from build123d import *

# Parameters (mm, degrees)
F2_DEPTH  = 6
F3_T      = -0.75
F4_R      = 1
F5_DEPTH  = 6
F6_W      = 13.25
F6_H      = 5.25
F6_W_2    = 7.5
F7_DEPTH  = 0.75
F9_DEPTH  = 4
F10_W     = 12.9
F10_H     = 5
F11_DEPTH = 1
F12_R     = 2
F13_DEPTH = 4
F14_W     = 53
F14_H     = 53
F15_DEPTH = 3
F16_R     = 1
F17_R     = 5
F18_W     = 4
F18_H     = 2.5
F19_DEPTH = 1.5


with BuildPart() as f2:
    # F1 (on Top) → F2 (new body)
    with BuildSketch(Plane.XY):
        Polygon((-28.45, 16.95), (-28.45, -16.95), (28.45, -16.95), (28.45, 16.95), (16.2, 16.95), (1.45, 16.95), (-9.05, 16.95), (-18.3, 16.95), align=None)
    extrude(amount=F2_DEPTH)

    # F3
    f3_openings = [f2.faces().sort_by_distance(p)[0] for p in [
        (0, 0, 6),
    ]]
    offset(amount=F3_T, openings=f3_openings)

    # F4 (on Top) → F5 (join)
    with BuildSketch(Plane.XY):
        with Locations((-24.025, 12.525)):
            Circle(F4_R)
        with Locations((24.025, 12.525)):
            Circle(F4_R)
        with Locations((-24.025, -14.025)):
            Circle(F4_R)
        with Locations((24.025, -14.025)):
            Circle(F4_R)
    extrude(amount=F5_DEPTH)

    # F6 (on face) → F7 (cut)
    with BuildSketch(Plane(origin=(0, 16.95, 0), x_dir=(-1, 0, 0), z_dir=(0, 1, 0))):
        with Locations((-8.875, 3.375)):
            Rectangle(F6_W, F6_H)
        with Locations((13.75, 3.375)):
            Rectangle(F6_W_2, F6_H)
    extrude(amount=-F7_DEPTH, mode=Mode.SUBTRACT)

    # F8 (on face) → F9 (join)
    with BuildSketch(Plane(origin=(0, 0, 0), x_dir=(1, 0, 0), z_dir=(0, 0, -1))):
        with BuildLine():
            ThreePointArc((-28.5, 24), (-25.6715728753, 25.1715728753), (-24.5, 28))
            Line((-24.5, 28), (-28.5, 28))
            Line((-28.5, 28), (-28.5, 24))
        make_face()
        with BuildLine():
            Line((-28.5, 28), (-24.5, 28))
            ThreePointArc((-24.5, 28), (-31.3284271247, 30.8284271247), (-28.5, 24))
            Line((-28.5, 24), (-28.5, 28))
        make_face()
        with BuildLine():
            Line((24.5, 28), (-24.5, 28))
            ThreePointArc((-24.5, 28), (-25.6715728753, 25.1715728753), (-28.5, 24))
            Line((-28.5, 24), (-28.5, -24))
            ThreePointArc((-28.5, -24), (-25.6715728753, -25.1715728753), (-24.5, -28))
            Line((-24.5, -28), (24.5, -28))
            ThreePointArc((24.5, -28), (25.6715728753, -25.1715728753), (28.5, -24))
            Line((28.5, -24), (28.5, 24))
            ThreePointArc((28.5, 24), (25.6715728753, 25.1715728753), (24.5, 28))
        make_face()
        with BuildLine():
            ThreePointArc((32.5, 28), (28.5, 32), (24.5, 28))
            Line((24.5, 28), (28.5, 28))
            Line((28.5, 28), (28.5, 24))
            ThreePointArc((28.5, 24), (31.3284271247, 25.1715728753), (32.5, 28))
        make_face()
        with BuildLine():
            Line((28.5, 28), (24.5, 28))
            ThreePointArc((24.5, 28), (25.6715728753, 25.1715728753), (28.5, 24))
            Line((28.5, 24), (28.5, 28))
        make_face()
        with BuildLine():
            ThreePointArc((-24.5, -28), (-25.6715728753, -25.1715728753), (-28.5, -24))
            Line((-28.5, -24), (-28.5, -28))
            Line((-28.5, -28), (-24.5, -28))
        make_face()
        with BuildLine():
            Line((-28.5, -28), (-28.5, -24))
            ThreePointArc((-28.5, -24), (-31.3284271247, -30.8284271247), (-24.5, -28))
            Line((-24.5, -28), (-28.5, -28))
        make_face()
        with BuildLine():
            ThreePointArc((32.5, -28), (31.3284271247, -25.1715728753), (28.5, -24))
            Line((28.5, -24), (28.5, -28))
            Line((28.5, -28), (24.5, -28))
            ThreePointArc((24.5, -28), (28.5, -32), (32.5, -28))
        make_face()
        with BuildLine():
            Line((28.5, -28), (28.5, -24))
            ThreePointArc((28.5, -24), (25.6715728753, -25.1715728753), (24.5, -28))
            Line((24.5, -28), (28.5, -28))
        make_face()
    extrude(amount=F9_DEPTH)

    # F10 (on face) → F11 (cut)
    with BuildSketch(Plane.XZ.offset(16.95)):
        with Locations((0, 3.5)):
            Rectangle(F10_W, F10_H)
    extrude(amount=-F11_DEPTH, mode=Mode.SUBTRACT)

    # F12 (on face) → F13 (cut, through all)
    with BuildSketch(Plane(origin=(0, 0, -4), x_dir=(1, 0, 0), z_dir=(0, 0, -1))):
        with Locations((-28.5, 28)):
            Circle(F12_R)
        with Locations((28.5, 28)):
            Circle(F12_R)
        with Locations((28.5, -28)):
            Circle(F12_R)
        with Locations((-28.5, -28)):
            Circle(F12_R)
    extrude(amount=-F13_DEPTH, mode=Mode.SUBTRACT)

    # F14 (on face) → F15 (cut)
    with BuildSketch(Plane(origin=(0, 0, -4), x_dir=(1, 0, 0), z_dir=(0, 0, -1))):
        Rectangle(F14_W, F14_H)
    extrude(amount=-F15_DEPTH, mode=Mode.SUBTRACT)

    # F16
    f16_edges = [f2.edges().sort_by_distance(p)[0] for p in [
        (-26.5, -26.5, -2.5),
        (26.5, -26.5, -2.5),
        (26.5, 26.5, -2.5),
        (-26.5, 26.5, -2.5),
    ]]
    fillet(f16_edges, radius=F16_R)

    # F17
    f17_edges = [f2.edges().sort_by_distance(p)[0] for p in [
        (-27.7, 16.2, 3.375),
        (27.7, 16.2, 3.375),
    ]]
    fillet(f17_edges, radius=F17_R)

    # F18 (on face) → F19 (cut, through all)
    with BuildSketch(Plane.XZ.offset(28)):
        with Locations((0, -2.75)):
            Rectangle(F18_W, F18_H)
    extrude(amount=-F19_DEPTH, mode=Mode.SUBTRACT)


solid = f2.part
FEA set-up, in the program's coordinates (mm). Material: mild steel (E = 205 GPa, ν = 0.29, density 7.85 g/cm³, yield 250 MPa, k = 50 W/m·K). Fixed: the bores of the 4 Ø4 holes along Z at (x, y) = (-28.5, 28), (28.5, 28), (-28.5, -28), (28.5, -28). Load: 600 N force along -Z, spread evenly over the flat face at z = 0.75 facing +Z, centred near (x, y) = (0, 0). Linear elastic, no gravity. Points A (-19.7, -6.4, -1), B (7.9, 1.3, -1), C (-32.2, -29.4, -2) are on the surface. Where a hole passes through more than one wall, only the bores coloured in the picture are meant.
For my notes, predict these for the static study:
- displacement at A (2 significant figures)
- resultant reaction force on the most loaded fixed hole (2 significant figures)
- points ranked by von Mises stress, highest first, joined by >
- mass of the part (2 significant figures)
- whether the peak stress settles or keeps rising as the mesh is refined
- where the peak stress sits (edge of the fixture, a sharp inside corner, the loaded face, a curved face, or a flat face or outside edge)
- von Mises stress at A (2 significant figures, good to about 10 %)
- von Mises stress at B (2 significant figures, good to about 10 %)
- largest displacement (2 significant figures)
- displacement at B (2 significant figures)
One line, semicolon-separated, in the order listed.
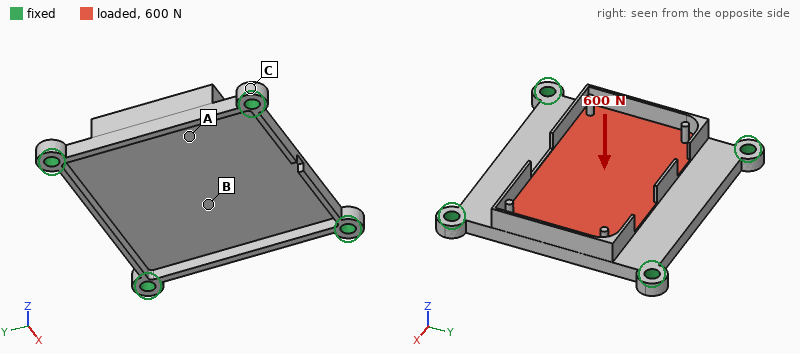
0.050 mm; 440 N; B > A > C; 54 g; keeps rising; a sharp inside corner; 34 MPa; 63 MPa; 0.11 mm; 0.100 mm
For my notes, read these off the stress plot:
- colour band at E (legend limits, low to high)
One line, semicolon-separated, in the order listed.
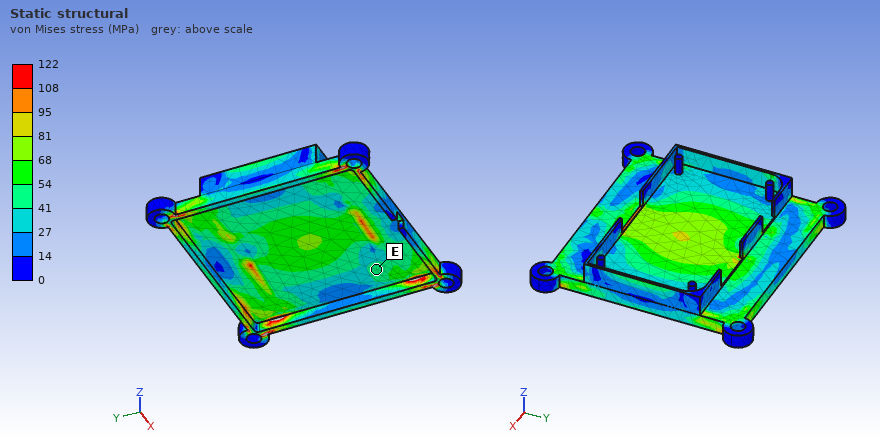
41 to 54 MPa
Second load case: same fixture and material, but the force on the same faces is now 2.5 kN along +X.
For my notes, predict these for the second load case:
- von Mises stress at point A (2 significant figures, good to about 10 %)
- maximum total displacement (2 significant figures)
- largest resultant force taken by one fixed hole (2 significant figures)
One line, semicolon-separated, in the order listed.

8.4 MPa; 7.7 µm; 700 N
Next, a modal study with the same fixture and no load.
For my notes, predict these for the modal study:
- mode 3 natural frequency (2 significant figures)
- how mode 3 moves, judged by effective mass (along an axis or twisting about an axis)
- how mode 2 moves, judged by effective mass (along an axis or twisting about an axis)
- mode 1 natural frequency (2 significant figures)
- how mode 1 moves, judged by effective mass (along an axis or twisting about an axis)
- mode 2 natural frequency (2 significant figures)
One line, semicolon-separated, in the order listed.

6000 Hz; twisting about Y; twisting about X; 2500 Hz; along Z; 4700 Hz
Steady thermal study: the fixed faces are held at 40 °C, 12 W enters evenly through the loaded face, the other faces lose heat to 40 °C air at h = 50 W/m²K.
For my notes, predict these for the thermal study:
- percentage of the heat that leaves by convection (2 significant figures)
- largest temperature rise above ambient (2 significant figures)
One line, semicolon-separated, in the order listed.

54 %; 28 K
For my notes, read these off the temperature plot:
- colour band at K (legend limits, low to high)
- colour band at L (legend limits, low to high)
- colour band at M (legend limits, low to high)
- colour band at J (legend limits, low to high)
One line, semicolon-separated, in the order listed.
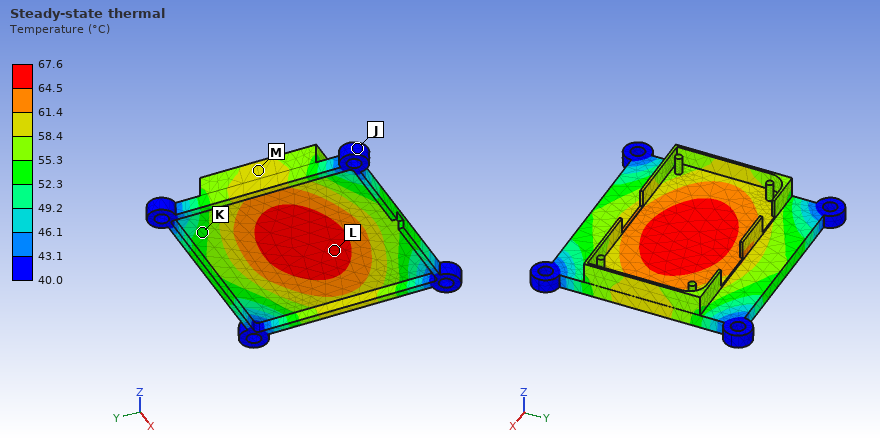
52.3 to 55.3 °C; 64.5 to 67.6 °C; 58.4 to 61.4 °C; 40.0 to 43.1 °C
